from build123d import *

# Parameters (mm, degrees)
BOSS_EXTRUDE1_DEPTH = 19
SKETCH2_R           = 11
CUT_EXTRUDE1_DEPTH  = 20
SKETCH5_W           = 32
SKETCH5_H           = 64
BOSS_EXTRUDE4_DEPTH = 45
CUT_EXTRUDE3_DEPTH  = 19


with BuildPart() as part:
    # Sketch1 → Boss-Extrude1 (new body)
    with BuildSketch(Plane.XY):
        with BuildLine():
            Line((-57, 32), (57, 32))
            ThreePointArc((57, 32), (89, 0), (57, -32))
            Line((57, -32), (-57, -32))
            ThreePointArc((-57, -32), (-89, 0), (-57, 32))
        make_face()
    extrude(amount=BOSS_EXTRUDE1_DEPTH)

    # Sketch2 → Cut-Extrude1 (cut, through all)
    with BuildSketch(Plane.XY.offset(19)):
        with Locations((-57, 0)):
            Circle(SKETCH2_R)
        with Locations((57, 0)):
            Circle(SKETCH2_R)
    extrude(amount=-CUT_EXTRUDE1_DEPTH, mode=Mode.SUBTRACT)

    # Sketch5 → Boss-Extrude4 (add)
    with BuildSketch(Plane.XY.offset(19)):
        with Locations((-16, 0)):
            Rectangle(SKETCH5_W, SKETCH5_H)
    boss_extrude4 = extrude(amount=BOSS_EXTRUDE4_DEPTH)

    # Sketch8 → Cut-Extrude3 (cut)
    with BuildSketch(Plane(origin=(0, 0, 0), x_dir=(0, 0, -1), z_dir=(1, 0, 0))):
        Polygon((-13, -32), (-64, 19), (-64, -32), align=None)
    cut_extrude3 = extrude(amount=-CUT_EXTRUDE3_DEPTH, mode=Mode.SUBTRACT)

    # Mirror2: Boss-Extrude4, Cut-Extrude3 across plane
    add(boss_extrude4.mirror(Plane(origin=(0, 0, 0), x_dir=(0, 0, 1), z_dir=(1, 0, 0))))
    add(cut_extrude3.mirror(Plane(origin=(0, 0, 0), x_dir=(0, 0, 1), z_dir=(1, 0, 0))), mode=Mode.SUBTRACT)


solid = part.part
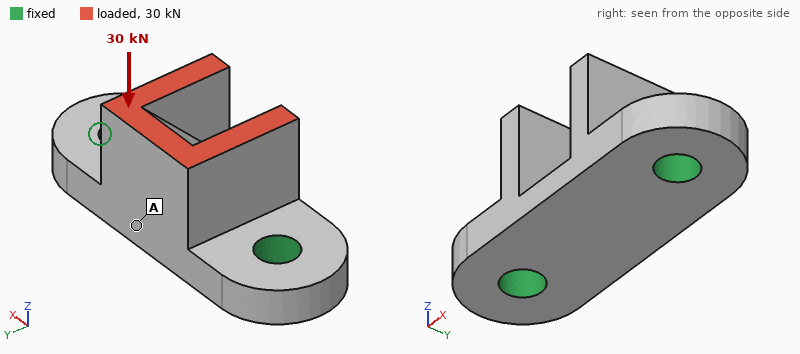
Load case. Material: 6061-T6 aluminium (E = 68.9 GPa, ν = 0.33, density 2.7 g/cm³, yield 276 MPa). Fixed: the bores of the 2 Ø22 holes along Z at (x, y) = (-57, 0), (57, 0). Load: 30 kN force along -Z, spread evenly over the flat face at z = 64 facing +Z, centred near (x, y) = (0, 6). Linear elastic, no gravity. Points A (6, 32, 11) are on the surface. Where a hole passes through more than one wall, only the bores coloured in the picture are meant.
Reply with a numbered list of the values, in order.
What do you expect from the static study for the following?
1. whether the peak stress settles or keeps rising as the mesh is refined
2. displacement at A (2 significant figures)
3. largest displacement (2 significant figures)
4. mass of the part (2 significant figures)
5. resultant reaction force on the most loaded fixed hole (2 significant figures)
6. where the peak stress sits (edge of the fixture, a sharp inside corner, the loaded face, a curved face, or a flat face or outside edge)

1. keeps rising
2. 50 µm
3. 64 µm
4. 860 g
5. 16 kN
6. edge of the fixture
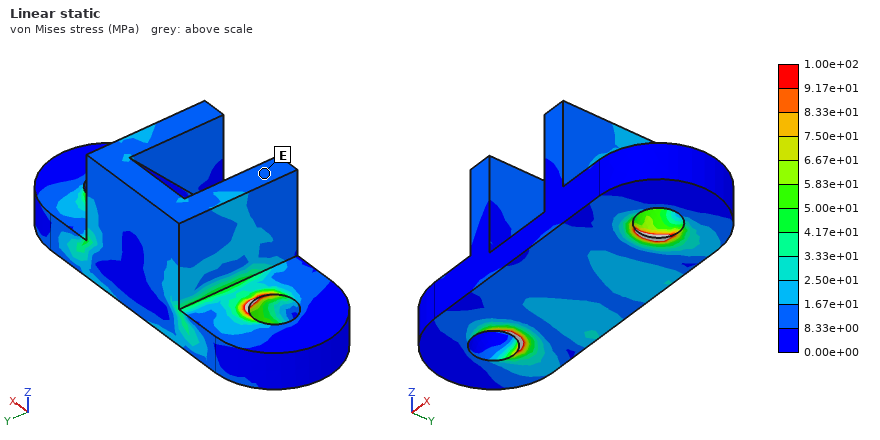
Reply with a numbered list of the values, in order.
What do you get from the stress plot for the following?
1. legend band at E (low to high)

1. 8.33e+00 to 1.67e+01 MPa
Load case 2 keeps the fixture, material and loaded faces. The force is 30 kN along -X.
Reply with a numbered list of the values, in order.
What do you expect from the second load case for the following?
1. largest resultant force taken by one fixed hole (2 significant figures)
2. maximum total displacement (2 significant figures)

1. 24 kN
2. 0.24 mm
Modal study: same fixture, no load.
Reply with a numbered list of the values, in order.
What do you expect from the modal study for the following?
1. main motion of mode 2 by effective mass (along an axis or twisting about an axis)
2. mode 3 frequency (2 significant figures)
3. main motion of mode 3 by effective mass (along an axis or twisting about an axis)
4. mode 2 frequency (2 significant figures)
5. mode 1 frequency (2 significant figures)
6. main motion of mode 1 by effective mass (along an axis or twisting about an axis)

1. along Z
2. 7000 Hz
3. along X
4. 6300 Hz
5. 3500 Hz
6. along Y
